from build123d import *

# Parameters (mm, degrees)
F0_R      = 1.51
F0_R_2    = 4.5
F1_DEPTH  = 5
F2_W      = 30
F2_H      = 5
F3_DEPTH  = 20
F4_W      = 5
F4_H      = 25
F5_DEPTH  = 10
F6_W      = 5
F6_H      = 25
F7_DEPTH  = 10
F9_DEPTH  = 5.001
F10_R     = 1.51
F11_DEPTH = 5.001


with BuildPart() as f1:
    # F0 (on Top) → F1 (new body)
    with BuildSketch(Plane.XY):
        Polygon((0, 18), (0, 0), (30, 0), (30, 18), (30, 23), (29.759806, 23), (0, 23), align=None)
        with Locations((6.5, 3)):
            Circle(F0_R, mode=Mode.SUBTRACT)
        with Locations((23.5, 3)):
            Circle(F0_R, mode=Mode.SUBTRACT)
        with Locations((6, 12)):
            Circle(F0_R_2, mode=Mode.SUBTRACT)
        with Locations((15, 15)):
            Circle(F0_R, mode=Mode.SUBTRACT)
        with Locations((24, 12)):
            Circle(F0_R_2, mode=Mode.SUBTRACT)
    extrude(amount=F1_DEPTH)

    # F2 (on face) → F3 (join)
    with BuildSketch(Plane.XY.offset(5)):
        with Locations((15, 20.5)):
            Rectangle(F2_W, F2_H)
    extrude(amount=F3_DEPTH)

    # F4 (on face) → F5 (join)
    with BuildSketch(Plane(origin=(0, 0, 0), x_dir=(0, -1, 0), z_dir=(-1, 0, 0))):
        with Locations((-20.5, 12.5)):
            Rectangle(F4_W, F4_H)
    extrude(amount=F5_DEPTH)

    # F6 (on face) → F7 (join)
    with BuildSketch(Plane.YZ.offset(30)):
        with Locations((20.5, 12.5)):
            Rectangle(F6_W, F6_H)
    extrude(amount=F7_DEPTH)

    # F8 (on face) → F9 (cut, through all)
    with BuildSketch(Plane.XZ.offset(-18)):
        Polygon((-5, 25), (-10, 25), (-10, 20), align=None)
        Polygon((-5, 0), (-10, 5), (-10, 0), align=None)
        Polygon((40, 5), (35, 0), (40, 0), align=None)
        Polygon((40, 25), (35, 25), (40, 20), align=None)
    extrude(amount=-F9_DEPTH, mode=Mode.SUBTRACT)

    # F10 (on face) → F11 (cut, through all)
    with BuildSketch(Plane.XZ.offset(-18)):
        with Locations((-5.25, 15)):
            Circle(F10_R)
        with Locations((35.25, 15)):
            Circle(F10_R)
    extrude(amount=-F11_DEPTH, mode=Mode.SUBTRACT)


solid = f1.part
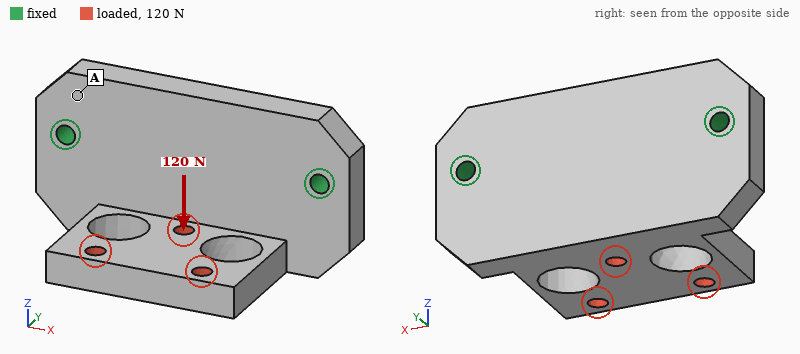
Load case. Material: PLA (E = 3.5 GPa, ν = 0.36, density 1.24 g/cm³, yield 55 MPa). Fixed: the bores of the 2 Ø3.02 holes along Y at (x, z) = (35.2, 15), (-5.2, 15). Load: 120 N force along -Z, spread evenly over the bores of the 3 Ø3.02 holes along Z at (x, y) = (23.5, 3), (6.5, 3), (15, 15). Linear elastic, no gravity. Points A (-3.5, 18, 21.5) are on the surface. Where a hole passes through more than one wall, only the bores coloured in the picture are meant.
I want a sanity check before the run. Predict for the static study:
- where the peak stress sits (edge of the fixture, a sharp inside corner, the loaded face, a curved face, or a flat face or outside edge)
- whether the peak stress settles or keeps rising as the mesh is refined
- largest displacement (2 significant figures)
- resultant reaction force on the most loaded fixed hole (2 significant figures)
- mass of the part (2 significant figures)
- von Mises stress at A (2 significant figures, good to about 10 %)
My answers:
edge of the fixture
keeps rising
0.68 mm
63 N
9.8 g
3.6 MPa
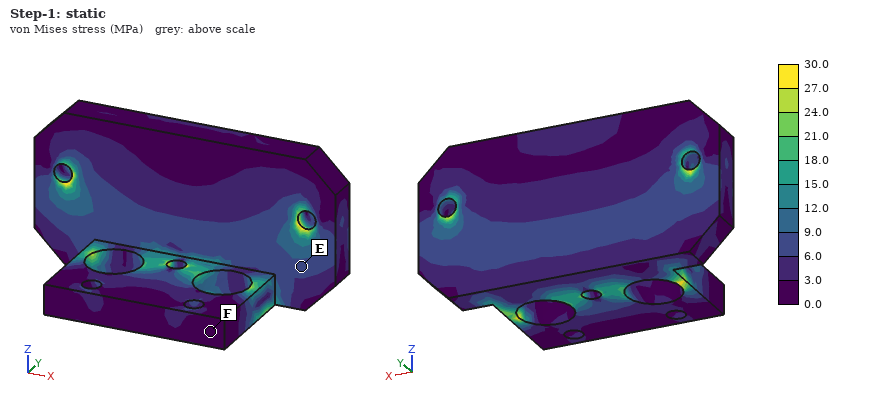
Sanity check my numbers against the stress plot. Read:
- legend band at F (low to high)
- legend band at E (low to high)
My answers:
0.0 to 3.0 MPa
6.0 to 9.0 MPa
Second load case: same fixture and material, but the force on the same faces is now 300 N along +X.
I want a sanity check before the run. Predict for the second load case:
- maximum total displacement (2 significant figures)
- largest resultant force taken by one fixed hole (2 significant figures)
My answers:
0.32 mm
210 N
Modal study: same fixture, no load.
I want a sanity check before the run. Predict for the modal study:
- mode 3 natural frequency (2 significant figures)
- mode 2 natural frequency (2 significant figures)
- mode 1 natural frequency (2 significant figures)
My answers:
3300 Hz
3200 Hz
1600 Hz
